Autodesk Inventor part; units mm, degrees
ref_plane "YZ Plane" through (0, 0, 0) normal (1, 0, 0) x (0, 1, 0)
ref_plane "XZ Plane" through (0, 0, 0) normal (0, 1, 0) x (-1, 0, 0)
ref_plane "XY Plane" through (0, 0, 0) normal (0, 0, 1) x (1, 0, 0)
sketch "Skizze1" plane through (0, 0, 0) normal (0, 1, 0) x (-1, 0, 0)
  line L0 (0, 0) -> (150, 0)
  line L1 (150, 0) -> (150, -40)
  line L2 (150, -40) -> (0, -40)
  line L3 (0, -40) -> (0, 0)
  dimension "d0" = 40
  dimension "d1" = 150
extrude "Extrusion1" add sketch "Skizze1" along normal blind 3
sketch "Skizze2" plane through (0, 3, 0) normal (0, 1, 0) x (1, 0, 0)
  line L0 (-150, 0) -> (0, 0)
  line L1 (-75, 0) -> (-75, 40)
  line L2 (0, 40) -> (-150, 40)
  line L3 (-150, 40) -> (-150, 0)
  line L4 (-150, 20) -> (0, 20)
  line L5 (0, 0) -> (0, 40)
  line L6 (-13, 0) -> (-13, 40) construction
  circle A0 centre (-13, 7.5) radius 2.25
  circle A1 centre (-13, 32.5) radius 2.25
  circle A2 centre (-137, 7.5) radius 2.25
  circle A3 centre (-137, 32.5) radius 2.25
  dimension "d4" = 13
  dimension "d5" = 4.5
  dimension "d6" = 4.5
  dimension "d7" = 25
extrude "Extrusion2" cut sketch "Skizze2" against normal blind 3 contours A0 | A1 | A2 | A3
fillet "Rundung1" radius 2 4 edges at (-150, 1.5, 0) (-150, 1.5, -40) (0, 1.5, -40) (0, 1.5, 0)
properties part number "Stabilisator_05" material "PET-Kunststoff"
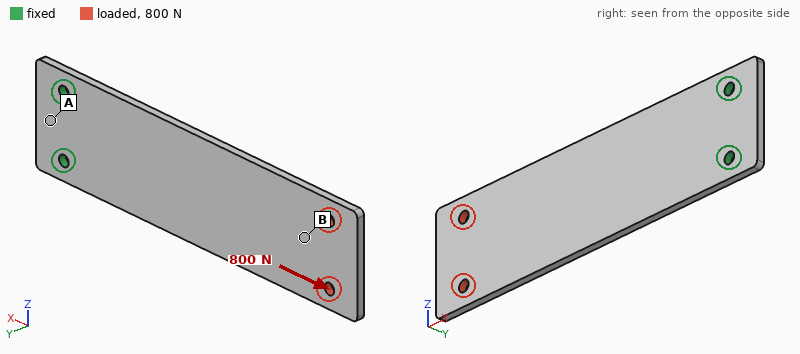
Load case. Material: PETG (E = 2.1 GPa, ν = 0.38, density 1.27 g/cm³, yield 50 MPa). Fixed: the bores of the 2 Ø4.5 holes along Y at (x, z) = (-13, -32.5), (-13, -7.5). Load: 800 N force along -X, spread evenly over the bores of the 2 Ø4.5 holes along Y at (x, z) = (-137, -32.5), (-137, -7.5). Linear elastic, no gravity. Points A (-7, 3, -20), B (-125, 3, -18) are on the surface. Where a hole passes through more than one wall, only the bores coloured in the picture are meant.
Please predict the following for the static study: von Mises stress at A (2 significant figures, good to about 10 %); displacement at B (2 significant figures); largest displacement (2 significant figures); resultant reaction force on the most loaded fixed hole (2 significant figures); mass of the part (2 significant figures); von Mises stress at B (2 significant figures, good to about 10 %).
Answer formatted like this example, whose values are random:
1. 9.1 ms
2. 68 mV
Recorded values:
1. 1.6 MPa
2. 0.36 mm
3. 0.43 mm
4. 400 N
5. 23 g
6. 5.5 MPa
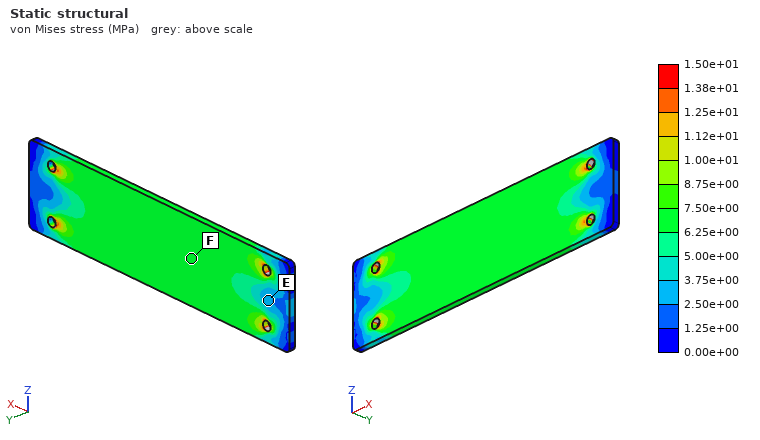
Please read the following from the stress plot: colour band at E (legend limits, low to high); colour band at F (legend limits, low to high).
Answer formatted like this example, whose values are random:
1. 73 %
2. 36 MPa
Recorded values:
1. 2.50e+00 to 3.75e+00 MPa
2. 6.25e+00 to 7.50e+00 MPa
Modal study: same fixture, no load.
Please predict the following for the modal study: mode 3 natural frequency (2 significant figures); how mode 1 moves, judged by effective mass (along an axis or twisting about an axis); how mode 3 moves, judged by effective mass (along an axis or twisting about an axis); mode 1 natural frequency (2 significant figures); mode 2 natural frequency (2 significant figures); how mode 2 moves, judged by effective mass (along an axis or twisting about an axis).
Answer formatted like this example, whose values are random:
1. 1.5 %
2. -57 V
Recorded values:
1. 230 Hz
2. along Y
3. twisting about X
4. 34 Hz
5. 210 Hz
6. along Y
